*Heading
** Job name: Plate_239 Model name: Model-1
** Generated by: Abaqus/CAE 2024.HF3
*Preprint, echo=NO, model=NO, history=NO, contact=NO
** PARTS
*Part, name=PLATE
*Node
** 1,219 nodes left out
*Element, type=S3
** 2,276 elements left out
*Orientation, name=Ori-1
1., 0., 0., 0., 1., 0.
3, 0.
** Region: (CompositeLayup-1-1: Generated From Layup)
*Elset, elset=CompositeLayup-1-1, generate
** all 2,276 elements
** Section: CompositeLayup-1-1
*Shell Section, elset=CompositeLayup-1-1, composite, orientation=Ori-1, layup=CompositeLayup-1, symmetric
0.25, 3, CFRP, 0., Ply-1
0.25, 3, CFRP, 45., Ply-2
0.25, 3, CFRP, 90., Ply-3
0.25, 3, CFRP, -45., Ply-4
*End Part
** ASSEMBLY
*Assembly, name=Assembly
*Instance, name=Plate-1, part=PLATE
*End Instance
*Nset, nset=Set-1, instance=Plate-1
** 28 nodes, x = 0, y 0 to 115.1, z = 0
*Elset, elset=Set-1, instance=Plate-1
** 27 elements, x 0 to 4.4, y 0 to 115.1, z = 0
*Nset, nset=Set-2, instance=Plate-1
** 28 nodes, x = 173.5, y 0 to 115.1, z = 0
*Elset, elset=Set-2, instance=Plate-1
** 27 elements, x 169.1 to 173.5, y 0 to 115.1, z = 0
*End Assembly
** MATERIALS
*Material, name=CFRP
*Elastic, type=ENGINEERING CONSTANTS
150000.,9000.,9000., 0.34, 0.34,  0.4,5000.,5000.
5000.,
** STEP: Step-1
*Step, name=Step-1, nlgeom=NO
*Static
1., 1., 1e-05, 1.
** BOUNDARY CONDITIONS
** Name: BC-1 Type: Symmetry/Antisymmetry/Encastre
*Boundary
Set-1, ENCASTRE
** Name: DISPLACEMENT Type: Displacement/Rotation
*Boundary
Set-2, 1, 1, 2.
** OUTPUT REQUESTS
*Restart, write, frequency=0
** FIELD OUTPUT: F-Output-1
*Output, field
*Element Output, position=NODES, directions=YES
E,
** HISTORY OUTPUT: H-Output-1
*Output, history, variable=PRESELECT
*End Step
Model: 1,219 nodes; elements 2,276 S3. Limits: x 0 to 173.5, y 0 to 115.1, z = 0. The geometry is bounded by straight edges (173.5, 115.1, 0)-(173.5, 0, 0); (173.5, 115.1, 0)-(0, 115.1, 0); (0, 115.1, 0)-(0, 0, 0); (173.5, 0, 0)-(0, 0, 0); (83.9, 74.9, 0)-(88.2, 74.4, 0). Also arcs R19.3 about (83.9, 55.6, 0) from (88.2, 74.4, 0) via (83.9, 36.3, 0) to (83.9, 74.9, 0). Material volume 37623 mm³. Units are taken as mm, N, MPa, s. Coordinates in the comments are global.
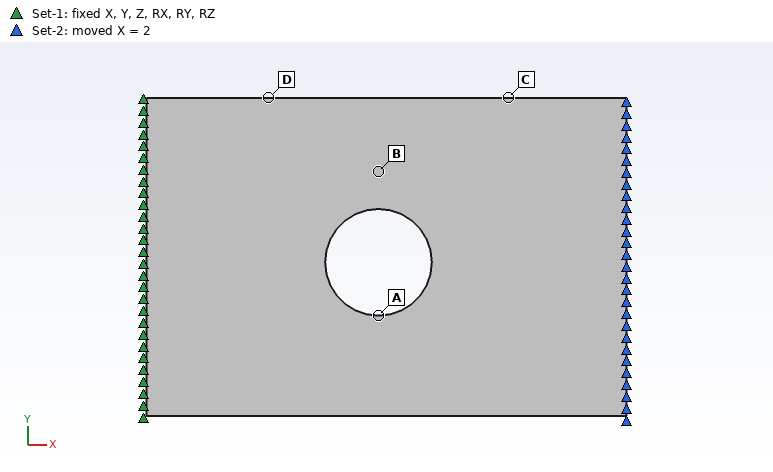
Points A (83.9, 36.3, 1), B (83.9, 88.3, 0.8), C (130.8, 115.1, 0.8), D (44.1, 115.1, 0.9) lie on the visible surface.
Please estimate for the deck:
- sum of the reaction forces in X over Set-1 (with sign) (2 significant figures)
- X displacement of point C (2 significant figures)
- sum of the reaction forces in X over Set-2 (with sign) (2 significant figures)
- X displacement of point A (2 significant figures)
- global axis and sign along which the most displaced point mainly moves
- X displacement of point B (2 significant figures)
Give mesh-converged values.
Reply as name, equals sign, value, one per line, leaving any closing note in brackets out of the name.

sum of the reaction forces in X over Set-1 (with sign) = -1.3e+05 N
X displacement of point C = 1.5 mm
sum of the reaction forces in X over Set-2 (with sign) = 1.3e+05 N
X displacement of point A = 0.96 mm
global axis and sign along which the most displaced point mainly moves = +X
X displacement of point B = 0.97 mm
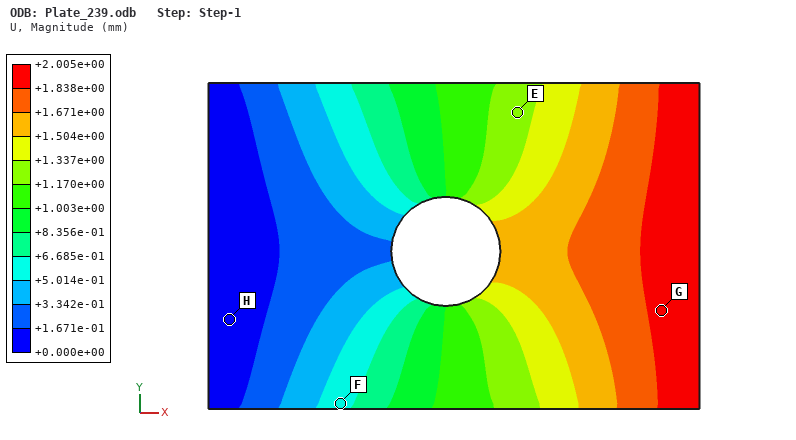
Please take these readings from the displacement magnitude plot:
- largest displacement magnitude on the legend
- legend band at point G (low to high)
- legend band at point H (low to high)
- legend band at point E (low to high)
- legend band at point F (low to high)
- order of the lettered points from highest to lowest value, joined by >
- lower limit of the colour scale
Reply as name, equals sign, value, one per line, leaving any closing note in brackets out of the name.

largest displacement magnitude on the legend = +2.005e+00 mm
legend band at point G = +1.838e+00 to +2.005e+00 mm
legend band at point H = +0.000e+00 to +1.671e-01 mm
legend band at point E = +1.170e+00 to +1.337e+00 mm
legend band at point F = +5.014e-01 to +6.685e-01 mm
order of the lettered points from highest to lowest value, joined by > = G > E > F > H
lower limit of the colour scale = +0.000e+00 mm
